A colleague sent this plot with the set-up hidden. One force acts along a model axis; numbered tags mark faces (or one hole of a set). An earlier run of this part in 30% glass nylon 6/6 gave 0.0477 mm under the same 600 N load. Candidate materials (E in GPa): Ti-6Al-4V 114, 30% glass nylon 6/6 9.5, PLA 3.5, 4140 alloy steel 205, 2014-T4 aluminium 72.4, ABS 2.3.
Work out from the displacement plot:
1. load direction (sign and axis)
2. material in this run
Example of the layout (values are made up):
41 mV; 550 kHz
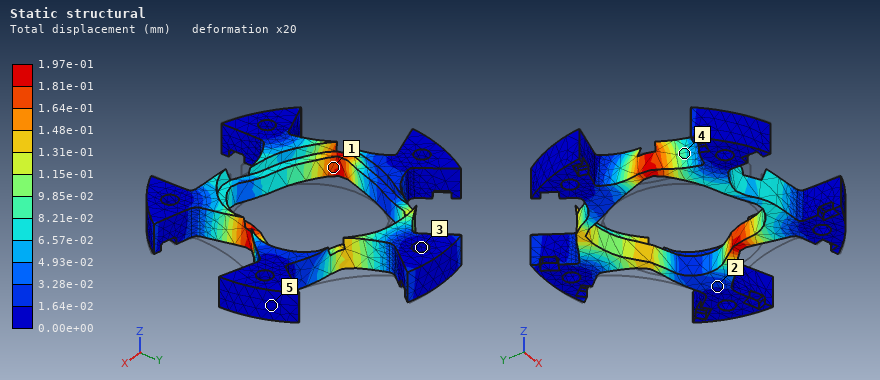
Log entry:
-X; ABS
